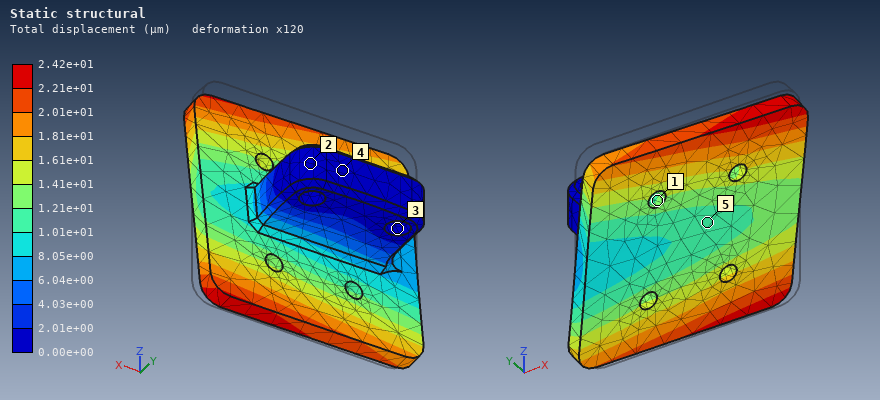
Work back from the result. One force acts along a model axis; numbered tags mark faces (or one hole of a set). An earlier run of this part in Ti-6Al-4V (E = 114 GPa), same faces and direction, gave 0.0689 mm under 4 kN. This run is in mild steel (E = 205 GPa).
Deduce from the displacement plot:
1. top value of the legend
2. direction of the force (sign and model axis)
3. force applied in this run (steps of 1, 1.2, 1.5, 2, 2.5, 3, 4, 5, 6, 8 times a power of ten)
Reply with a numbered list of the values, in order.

1. 2.42e+01 µm
2. -Z
3. 2.5 kN
